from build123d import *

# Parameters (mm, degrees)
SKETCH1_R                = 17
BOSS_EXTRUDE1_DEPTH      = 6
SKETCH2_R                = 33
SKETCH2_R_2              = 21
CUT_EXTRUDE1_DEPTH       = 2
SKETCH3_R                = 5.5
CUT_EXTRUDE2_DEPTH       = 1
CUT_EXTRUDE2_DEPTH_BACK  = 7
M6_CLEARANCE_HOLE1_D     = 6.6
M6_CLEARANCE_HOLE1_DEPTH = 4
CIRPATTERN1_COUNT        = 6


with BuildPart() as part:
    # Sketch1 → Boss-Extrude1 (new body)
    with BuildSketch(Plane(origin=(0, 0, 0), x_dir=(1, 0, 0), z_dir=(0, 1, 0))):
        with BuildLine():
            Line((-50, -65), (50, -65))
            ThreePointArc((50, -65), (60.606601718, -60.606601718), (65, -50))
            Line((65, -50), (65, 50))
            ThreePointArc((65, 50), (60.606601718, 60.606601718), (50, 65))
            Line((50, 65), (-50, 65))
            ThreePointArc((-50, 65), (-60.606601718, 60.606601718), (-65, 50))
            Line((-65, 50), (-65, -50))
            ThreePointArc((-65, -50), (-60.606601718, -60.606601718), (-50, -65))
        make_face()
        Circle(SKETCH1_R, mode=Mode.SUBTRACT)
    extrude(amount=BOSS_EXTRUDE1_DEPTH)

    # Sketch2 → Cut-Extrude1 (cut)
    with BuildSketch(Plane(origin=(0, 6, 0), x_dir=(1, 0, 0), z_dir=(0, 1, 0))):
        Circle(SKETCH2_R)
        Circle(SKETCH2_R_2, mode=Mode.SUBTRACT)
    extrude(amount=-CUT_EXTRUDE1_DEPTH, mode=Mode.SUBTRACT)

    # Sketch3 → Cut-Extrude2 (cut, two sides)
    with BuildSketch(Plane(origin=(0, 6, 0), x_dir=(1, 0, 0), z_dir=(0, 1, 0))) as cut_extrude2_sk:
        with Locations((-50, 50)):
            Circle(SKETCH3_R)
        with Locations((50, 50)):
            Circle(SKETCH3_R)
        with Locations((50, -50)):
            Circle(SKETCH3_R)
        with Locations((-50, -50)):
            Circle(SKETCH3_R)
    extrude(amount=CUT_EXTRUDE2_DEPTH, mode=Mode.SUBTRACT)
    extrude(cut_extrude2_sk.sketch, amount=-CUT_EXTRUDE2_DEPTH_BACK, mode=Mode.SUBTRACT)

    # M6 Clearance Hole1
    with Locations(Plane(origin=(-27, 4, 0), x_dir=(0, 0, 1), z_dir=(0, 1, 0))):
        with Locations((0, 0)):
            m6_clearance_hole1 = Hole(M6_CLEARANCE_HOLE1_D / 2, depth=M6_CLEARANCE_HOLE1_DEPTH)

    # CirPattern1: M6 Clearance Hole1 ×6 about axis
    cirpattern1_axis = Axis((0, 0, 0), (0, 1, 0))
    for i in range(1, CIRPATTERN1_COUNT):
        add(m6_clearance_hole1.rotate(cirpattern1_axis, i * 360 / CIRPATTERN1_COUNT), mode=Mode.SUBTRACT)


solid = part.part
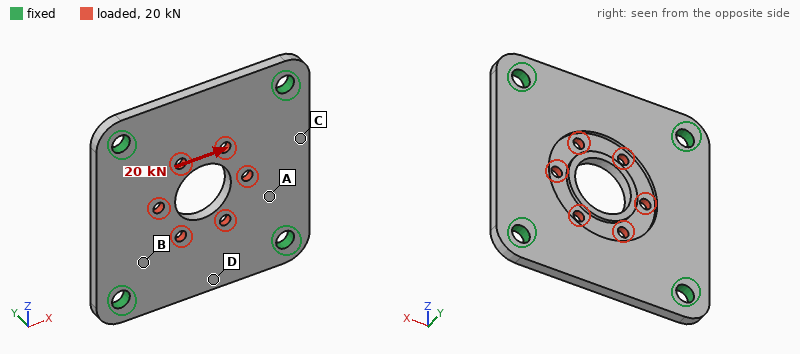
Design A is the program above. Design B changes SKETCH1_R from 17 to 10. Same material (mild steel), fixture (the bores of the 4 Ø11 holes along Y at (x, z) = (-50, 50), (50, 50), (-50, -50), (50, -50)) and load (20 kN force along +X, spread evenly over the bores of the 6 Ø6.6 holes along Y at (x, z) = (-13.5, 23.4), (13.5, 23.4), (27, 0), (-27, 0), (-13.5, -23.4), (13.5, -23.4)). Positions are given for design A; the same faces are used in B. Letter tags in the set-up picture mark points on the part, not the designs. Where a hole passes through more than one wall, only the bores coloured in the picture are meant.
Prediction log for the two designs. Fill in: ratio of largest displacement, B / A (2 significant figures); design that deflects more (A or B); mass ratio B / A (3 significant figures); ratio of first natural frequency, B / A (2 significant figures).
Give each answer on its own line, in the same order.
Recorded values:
0.91
A
1.04
0.94
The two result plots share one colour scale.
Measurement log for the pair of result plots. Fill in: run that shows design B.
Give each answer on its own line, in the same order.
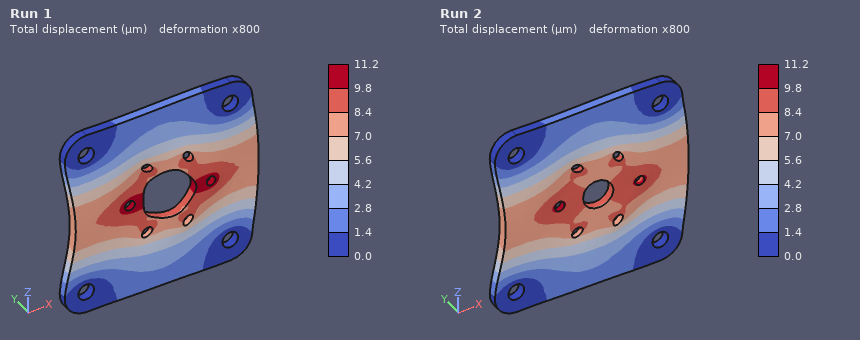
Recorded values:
Run 2
